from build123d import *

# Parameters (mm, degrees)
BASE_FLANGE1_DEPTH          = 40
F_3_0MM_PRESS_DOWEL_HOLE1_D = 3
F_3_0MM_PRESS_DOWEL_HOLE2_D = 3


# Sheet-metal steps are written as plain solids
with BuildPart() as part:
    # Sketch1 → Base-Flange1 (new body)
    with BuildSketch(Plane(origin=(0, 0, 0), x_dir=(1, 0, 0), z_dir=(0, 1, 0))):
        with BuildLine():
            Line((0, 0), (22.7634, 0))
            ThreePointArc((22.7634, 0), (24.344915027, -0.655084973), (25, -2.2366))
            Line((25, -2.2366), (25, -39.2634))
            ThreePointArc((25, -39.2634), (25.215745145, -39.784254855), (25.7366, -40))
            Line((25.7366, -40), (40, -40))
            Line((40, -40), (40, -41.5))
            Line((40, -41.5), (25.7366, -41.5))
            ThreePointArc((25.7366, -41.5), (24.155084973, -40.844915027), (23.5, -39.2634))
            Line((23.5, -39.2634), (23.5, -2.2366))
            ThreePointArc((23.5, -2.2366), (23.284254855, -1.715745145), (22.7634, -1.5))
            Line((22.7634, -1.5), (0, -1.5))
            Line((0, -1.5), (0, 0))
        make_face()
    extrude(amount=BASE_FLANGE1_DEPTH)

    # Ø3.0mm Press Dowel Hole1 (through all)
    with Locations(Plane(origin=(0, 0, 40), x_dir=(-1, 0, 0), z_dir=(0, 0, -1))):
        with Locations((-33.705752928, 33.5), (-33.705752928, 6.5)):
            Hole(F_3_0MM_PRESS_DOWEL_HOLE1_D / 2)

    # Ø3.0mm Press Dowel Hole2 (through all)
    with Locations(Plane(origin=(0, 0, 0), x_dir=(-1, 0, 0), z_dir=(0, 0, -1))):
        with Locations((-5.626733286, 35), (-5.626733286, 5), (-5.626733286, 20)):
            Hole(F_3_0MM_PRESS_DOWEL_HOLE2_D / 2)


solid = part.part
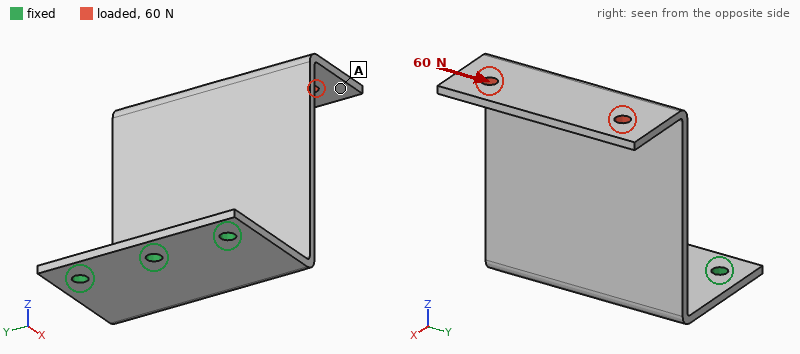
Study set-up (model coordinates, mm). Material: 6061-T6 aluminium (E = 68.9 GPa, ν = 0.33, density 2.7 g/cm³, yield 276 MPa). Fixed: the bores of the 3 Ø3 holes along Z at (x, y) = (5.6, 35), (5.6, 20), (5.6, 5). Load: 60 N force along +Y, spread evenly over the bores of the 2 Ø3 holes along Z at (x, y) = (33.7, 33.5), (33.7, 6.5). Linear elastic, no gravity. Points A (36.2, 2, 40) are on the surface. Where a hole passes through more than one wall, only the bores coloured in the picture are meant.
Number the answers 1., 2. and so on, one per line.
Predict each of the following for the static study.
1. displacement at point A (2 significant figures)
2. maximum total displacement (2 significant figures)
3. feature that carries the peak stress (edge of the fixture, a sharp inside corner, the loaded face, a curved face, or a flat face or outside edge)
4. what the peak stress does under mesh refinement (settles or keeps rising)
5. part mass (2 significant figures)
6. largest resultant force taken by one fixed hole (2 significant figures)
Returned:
1. 0.59 mm
2. 0.64 mm
3. edge of the fixture
4. keeps rising
5. 13 g
6. 96 N
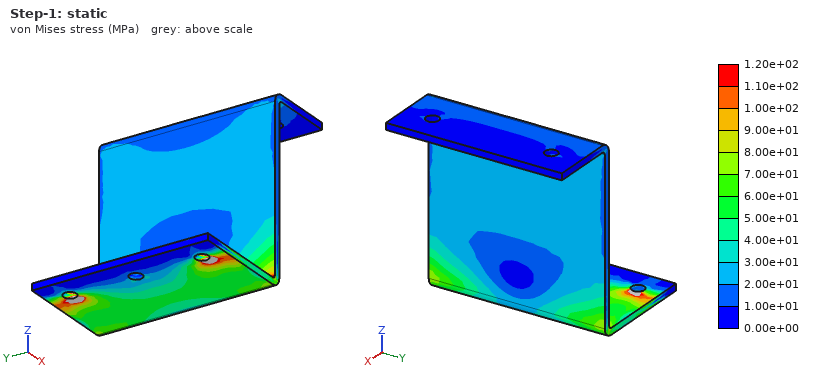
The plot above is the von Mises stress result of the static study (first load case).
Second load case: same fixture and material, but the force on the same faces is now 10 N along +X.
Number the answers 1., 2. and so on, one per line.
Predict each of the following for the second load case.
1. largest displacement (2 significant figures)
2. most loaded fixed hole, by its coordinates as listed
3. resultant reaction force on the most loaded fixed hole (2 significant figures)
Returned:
1. 0.70 mm
2. (5.6, 20)
3. 5.9 N
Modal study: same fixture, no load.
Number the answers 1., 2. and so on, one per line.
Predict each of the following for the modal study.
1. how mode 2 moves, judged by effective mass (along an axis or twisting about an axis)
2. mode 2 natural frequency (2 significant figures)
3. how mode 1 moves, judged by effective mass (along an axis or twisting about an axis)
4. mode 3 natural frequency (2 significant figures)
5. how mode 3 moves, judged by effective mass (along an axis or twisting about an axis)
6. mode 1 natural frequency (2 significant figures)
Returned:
1. along Y
2. 750 Hz
3. along X
4. 1100 Hz
5. twisting about Z
6. 300 Hz
